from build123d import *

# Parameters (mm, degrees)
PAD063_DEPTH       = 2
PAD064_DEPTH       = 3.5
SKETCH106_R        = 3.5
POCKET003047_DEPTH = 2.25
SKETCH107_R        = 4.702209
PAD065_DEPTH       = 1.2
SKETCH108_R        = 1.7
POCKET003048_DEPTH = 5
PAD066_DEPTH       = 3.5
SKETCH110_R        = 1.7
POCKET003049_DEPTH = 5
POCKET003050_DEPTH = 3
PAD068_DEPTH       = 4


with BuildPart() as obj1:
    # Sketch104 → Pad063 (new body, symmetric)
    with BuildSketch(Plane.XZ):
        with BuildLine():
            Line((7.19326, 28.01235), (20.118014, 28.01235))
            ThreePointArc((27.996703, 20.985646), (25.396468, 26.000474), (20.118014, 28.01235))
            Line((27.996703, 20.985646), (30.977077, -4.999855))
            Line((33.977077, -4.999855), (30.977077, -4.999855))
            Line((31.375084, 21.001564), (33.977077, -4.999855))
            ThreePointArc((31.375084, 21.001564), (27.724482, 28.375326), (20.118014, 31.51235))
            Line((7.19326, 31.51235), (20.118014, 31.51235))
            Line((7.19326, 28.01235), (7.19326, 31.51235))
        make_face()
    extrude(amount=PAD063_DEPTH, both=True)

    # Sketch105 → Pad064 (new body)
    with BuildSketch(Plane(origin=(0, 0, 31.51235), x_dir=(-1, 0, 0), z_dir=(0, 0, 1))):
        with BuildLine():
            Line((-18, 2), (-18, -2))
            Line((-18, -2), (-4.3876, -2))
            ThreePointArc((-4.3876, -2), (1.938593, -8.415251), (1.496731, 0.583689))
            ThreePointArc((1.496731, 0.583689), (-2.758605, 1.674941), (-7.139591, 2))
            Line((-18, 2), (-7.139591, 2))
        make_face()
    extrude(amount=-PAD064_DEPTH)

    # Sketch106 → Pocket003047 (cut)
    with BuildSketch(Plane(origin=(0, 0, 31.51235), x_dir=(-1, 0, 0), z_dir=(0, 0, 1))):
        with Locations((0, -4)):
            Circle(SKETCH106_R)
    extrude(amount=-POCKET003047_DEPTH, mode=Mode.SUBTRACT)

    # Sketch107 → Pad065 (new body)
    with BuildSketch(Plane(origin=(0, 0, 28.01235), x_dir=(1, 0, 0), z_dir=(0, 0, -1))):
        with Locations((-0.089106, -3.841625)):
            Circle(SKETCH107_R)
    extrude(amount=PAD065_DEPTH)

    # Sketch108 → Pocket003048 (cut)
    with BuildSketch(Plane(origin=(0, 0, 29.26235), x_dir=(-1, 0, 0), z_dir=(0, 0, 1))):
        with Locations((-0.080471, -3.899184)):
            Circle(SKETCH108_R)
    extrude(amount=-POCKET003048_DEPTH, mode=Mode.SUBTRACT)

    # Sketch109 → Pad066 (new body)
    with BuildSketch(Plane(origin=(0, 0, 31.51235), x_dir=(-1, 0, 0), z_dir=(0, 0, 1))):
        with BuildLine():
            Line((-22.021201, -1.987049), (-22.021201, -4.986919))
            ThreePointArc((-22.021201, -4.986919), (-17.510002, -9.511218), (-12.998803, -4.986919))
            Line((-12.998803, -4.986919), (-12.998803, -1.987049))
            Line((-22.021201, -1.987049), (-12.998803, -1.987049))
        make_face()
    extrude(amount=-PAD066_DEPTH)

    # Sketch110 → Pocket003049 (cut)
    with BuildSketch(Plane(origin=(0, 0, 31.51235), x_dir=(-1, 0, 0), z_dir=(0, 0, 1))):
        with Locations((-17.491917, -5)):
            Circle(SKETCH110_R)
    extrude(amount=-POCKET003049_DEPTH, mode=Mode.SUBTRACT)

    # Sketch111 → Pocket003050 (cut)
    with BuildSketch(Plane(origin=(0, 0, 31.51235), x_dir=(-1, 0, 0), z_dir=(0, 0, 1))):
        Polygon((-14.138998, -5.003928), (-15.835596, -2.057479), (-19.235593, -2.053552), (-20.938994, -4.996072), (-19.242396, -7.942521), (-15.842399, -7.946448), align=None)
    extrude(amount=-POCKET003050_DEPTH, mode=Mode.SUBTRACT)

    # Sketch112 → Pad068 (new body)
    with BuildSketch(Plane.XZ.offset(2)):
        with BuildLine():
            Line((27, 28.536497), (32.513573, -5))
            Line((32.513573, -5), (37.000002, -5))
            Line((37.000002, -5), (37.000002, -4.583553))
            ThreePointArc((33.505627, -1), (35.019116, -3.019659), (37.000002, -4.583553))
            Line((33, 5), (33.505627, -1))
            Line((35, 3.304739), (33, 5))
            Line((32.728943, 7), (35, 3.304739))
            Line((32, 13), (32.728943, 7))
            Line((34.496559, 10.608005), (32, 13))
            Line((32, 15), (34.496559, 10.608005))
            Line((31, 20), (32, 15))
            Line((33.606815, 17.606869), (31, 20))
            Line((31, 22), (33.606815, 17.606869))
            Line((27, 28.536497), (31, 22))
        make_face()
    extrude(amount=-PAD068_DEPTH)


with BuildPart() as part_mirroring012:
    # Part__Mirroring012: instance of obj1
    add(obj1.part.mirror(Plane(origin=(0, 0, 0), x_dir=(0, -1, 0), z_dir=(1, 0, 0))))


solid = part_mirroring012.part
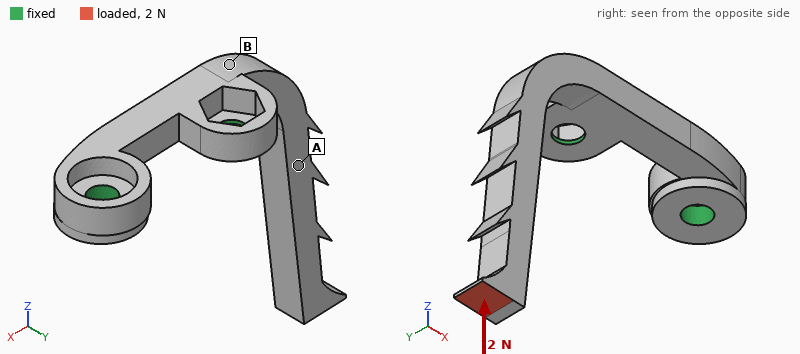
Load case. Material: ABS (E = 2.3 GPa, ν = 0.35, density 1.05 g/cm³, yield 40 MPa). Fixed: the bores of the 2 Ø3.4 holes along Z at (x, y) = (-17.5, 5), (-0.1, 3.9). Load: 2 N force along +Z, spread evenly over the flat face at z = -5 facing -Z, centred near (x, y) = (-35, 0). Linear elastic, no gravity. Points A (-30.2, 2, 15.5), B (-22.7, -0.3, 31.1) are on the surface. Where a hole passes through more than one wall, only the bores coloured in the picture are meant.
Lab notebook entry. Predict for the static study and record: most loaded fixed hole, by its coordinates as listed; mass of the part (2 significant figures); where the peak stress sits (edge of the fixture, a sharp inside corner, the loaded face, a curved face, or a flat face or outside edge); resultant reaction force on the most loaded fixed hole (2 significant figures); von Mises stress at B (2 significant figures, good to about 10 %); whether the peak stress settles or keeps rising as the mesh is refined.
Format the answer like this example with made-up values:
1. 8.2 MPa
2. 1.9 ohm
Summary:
1. (-17.5, 5)
2. 1.2 g
3. edge of the fixture
4. 4.5 N
5. 2.7 MPa
6. keeps rising
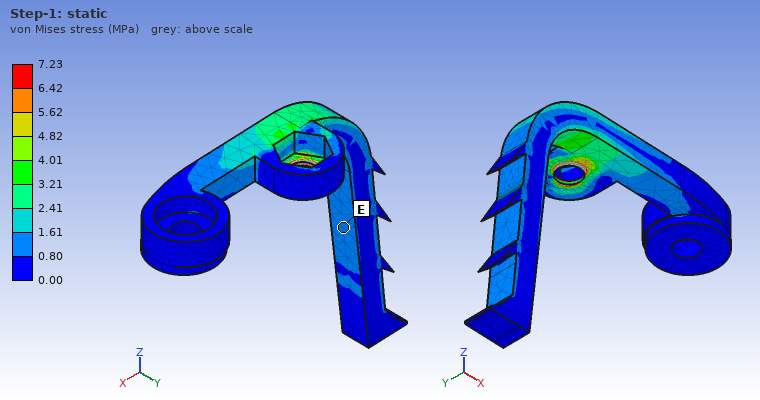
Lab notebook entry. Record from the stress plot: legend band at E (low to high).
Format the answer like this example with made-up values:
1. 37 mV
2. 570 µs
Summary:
1. 0.80 to 1.61 MPa
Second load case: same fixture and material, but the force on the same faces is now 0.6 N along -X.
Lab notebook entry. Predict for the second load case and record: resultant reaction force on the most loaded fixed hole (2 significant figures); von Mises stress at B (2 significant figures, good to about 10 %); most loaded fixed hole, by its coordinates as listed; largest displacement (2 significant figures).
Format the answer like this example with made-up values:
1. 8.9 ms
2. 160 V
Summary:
1. 2.2 N
2. 2.2 MPa
3. (-17.5, 5)
4. 0.58 mm
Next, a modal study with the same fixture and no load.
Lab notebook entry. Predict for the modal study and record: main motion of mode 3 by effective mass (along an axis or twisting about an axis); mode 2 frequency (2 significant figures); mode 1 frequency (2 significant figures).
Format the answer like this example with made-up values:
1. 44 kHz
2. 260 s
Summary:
1. along Z
2. 430 Hz
3. 380 Hz
